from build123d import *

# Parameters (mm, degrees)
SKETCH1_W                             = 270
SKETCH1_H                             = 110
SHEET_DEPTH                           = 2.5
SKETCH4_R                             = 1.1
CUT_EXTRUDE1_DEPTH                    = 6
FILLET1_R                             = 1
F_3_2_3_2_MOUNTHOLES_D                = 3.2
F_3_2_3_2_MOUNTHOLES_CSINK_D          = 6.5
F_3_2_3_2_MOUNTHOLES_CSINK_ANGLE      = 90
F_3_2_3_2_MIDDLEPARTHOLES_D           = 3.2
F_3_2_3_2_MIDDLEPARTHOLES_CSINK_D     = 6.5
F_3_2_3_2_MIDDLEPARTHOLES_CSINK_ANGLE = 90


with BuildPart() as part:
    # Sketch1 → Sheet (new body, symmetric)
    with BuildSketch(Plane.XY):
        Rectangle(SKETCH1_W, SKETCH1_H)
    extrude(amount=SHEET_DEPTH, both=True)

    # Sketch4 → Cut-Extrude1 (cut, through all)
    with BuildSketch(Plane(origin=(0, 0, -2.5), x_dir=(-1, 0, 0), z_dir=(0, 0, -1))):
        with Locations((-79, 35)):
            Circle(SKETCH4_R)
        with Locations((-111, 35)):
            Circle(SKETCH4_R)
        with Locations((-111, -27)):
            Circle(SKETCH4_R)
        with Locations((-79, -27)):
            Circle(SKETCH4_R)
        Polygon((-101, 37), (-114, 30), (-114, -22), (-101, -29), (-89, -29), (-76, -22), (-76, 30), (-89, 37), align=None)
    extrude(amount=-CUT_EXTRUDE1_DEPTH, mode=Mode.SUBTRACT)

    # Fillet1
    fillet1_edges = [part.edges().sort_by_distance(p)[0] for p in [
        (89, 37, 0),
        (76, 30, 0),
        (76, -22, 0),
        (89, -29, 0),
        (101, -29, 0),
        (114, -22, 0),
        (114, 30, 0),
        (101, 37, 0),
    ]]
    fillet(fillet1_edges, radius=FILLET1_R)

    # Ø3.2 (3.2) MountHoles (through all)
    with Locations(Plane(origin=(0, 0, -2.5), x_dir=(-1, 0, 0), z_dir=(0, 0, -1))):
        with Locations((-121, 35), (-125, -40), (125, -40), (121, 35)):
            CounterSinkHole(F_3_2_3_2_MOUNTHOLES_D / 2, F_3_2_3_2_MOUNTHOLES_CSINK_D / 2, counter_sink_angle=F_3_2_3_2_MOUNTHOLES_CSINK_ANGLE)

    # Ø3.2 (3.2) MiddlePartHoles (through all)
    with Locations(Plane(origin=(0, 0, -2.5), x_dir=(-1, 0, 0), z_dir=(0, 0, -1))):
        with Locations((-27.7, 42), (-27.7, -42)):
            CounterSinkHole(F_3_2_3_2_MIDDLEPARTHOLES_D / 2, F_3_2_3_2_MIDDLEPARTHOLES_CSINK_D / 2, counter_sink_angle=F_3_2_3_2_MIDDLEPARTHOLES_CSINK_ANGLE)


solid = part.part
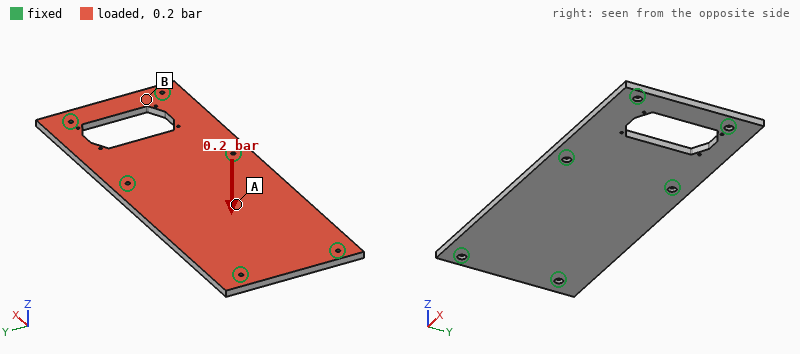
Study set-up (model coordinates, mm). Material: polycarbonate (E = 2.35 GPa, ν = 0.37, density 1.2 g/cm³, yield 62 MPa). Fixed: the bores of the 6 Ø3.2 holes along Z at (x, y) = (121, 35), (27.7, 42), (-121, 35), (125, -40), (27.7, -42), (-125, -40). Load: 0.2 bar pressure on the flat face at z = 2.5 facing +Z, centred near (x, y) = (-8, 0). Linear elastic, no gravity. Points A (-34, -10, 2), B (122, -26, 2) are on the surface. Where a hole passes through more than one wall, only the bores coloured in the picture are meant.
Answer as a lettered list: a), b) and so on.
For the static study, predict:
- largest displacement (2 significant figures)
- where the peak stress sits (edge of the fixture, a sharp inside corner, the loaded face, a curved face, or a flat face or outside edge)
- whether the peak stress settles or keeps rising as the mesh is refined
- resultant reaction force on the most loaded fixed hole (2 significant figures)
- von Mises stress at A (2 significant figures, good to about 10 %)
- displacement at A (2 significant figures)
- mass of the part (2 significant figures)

a) 1.8 mm
b) edge of the fixture
c) keeps rising
d) 160 N
e) 4.3 MPa
f) 1.6 mm
g) 160 g
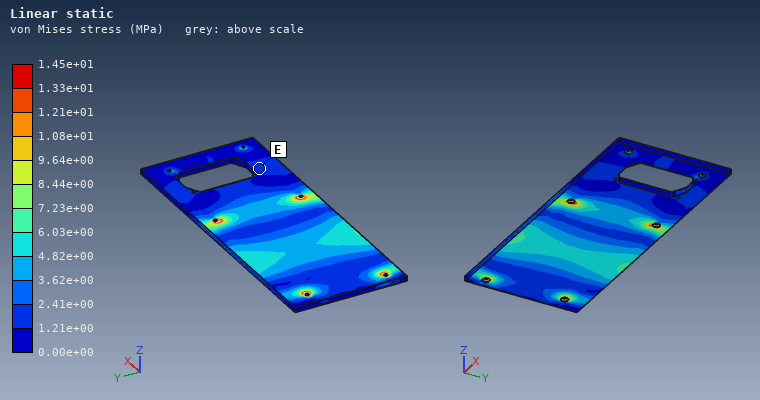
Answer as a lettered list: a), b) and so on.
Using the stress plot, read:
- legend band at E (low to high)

a) 1.21e+00 to 2.41e+00 MPa
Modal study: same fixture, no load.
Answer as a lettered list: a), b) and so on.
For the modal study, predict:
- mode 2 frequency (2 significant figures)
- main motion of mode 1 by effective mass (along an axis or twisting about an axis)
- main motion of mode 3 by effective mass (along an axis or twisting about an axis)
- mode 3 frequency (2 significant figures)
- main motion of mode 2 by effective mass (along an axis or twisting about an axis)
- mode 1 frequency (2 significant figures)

a) 380 Hz
b) along Z
c) along Z
d) 520 Hz
e) twisting about X
f) 250 Hz
